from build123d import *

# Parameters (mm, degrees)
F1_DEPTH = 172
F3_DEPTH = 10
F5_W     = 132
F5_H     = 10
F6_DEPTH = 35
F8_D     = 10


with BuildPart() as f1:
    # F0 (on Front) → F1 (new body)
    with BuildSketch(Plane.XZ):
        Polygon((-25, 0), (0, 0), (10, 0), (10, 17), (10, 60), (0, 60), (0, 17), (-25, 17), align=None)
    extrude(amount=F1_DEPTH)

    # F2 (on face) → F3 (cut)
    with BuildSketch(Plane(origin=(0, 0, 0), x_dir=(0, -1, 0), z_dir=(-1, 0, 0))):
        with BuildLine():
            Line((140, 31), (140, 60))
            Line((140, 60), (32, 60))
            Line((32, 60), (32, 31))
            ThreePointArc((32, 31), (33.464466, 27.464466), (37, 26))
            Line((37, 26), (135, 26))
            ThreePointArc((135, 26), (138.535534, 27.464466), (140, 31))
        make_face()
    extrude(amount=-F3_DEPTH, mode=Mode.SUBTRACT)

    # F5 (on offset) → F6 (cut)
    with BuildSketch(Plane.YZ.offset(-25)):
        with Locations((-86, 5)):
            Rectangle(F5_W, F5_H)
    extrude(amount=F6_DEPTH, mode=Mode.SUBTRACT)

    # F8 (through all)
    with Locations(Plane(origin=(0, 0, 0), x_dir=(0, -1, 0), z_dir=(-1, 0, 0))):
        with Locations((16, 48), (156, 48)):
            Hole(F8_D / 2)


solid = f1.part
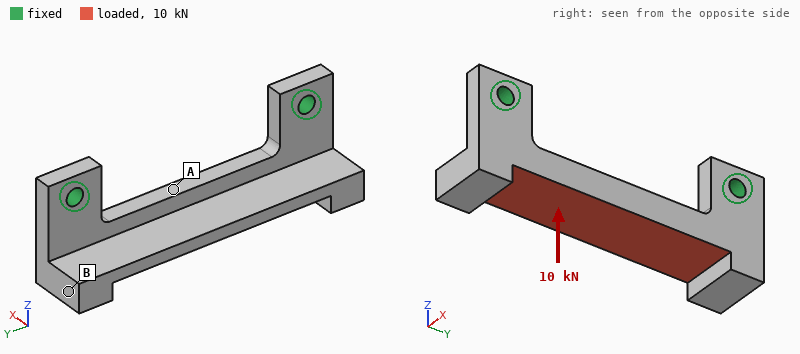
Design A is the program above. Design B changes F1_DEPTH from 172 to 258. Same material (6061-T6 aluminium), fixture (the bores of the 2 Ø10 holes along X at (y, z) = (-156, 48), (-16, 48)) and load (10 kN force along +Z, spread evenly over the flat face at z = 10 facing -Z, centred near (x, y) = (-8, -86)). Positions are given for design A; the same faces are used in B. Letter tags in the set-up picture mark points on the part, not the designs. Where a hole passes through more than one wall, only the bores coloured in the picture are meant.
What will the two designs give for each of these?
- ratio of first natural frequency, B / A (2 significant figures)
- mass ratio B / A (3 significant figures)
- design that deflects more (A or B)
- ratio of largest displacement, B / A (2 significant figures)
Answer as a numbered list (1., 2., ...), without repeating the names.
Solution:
1. 0.53
2. 1.96
3. A
4. 0.92
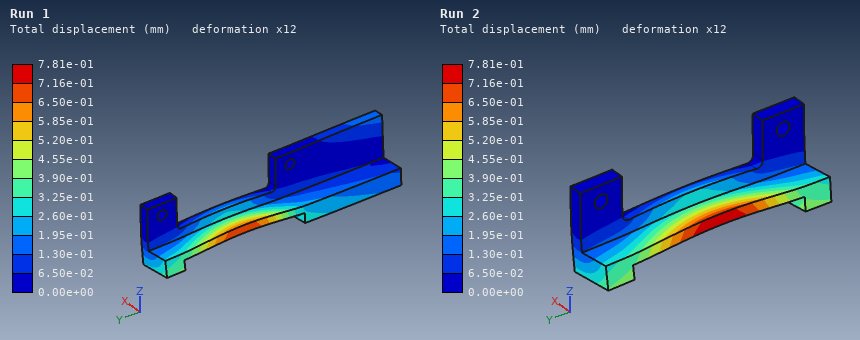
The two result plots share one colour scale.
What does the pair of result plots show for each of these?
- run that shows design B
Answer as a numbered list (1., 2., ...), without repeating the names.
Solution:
1. Run 1
